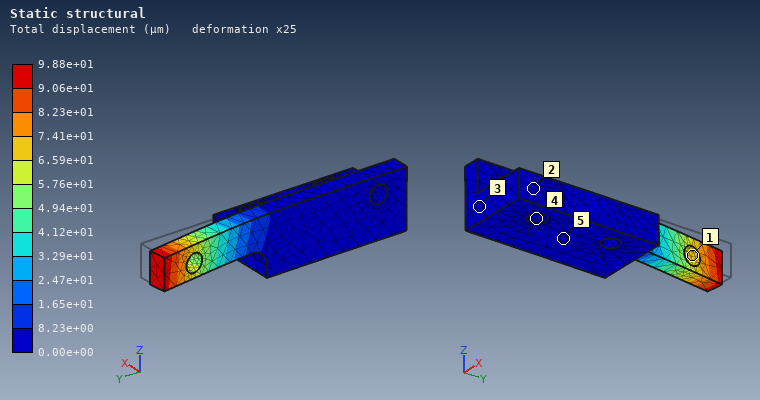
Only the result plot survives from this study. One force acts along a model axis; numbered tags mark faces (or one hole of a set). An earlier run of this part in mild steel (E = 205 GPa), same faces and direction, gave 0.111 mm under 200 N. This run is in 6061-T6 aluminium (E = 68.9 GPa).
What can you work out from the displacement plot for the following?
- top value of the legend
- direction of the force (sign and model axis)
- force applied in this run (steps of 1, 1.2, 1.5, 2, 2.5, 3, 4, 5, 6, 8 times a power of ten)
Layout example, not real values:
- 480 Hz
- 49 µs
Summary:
- 9.88e+01 µm
- -X
- 60 N
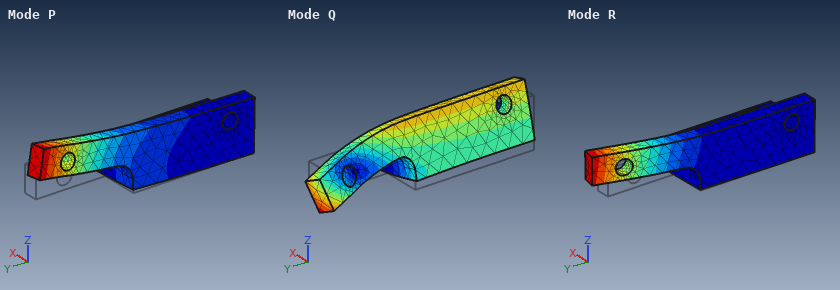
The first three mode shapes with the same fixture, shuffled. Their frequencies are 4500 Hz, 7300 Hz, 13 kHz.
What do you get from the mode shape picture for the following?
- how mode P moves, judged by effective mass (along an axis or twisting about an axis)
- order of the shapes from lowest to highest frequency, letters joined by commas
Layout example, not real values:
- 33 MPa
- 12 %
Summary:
- along Z
- R, P, Q
